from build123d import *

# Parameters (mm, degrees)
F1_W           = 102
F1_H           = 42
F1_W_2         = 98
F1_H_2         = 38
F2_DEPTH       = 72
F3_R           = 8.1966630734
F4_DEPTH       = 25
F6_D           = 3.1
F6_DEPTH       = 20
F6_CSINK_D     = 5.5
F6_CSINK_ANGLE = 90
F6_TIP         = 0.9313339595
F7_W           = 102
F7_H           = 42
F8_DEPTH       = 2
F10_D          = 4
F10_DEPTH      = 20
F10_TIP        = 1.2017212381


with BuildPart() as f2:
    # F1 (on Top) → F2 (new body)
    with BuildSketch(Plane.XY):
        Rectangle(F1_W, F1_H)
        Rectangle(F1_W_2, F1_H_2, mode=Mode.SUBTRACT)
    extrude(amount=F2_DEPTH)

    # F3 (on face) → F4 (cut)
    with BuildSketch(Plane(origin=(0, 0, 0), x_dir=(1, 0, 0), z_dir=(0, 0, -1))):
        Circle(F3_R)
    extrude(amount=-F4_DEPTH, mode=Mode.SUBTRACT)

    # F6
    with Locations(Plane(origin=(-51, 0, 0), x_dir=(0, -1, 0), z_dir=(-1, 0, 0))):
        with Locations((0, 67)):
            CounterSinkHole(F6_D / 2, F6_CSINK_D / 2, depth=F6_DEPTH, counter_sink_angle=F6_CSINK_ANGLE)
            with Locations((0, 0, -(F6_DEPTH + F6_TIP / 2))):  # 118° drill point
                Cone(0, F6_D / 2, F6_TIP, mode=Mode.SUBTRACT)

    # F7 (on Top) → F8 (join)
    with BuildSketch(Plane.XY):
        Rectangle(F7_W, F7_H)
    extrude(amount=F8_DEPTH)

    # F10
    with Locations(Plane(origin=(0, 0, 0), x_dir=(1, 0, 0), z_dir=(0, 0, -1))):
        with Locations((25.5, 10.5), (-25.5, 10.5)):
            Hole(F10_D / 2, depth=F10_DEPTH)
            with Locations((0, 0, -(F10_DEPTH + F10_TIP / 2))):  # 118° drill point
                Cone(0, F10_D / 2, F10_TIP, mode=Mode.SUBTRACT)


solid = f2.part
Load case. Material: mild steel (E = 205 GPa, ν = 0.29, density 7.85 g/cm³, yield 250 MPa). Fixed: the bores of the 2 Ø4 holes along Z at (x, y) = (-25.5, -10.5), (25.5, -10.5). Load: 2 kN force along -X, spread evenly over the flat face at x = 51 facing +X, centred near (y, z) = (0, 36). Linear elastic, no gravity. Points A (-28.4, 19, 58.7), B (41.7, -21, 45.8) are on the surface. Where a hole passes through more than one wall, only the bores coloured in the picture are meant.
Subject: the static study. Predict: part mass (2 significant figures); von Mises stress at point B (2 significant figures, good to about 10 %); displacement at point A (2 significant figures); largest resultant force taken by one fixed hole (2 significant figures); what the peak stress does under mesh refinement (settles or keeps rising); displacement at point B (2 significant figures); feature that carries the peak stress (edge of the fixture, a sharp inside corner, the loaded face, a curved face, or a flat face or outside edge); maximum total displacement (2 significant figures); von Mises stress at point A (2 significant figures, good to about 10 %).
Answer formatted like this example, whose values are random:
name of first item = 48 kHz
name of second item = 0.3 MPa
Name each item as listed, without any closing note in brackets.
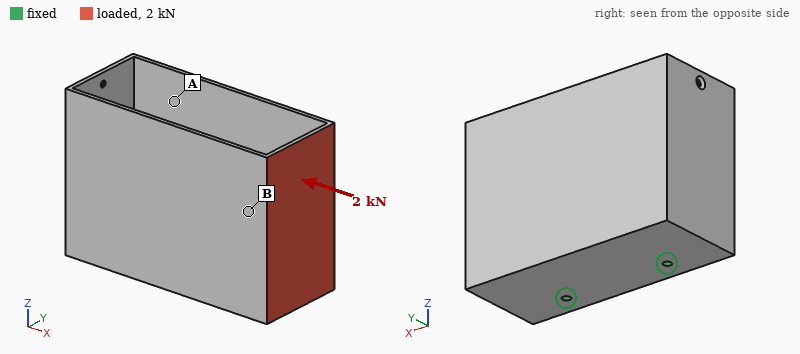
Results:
part mass = 370 g
von Mises stress at point B = 68 MPa
displacement at point A = 0.27 mm
largest resultant force taken by one fixed hole = 1.7 kN
what the peak stress does under mesh refinement = keeps rising
displacement at point B = 0.15 mm
feature that carries the peak stress = edge of the fixture
maximum total displacement = 0.35 mm
von Mises stress at point A = 24 MPa
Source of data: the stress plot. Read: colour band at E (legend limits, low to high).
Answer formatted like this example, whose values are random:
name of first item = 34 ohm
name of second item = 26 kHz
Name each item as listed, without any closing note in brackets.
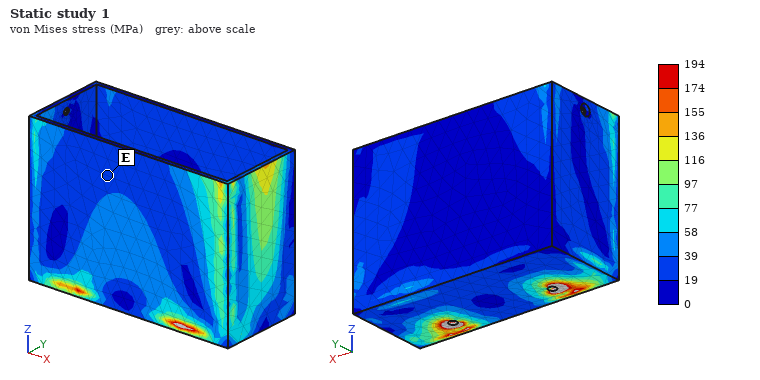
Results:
colour band at E = 19 to 39 MPa
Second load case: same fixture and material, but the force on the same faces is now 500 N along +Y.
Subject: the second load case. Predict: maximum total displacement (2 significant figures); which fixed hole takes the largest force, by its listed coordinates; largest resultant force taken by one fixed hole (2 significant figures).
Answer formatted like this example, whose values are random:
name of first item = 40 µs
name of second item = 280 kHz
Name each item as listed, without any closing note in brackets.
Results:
maximum total displacement = 0.87 mm
which fixed hole takes the largest force, by its listed coordinates = (25.5, -10.5)
largest resultant force taken by one fixed hole = 740 N
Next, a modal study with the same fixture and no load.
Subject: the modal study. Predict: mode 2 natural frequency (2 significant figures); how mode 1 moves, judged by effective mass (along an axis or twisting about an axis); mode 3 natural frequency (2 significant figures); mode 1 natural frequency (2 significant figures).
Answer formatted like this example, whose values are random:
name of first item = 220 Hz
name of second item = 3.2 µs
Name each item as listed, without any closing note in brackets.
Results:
mode 2 natural frequency = 600 Hz
how mode 1 moves, judged by effective mass = along Y
mode 3 natural frequency = 940 Hz
mode 1 natural frequency = 260 Hz
